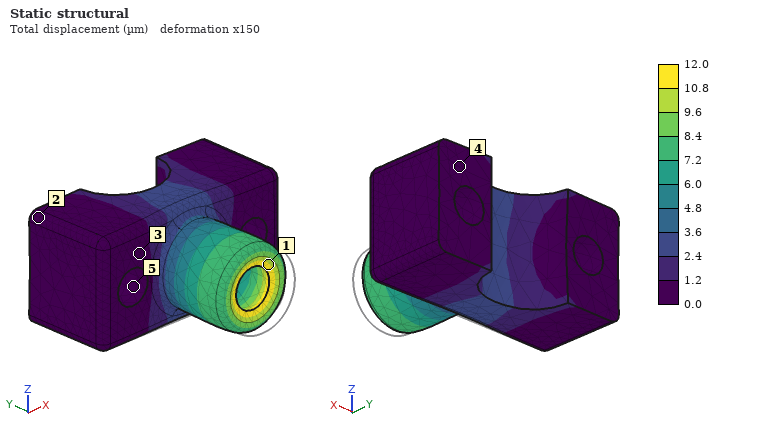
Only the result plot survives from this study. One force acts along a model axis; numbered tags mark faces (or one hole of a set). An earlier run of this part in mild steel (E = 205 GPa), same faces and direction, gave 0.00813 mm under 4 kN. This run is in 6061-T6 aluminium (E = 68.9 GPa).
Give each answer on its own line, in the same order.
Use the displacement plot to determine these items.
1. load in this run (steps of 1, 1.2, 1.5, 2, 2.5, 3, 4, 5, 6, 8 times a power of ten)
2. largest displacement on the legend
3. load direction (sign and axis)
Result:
2 kN
12.0 µm
+Y
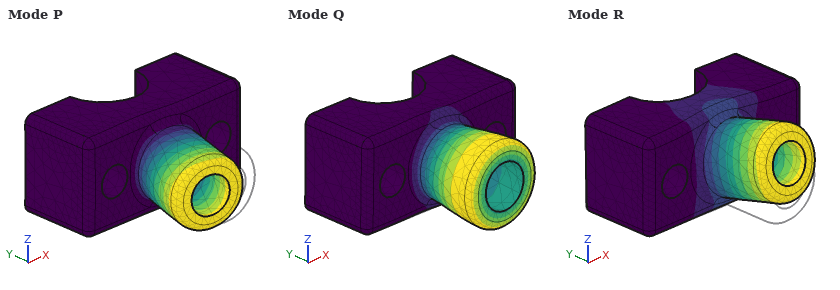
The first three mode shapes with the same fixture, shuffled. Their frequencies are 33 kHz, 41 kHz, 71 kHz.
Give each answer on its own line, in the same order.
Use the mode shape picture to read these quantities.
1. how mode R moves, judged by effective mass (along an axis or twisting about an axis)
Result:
along Z
